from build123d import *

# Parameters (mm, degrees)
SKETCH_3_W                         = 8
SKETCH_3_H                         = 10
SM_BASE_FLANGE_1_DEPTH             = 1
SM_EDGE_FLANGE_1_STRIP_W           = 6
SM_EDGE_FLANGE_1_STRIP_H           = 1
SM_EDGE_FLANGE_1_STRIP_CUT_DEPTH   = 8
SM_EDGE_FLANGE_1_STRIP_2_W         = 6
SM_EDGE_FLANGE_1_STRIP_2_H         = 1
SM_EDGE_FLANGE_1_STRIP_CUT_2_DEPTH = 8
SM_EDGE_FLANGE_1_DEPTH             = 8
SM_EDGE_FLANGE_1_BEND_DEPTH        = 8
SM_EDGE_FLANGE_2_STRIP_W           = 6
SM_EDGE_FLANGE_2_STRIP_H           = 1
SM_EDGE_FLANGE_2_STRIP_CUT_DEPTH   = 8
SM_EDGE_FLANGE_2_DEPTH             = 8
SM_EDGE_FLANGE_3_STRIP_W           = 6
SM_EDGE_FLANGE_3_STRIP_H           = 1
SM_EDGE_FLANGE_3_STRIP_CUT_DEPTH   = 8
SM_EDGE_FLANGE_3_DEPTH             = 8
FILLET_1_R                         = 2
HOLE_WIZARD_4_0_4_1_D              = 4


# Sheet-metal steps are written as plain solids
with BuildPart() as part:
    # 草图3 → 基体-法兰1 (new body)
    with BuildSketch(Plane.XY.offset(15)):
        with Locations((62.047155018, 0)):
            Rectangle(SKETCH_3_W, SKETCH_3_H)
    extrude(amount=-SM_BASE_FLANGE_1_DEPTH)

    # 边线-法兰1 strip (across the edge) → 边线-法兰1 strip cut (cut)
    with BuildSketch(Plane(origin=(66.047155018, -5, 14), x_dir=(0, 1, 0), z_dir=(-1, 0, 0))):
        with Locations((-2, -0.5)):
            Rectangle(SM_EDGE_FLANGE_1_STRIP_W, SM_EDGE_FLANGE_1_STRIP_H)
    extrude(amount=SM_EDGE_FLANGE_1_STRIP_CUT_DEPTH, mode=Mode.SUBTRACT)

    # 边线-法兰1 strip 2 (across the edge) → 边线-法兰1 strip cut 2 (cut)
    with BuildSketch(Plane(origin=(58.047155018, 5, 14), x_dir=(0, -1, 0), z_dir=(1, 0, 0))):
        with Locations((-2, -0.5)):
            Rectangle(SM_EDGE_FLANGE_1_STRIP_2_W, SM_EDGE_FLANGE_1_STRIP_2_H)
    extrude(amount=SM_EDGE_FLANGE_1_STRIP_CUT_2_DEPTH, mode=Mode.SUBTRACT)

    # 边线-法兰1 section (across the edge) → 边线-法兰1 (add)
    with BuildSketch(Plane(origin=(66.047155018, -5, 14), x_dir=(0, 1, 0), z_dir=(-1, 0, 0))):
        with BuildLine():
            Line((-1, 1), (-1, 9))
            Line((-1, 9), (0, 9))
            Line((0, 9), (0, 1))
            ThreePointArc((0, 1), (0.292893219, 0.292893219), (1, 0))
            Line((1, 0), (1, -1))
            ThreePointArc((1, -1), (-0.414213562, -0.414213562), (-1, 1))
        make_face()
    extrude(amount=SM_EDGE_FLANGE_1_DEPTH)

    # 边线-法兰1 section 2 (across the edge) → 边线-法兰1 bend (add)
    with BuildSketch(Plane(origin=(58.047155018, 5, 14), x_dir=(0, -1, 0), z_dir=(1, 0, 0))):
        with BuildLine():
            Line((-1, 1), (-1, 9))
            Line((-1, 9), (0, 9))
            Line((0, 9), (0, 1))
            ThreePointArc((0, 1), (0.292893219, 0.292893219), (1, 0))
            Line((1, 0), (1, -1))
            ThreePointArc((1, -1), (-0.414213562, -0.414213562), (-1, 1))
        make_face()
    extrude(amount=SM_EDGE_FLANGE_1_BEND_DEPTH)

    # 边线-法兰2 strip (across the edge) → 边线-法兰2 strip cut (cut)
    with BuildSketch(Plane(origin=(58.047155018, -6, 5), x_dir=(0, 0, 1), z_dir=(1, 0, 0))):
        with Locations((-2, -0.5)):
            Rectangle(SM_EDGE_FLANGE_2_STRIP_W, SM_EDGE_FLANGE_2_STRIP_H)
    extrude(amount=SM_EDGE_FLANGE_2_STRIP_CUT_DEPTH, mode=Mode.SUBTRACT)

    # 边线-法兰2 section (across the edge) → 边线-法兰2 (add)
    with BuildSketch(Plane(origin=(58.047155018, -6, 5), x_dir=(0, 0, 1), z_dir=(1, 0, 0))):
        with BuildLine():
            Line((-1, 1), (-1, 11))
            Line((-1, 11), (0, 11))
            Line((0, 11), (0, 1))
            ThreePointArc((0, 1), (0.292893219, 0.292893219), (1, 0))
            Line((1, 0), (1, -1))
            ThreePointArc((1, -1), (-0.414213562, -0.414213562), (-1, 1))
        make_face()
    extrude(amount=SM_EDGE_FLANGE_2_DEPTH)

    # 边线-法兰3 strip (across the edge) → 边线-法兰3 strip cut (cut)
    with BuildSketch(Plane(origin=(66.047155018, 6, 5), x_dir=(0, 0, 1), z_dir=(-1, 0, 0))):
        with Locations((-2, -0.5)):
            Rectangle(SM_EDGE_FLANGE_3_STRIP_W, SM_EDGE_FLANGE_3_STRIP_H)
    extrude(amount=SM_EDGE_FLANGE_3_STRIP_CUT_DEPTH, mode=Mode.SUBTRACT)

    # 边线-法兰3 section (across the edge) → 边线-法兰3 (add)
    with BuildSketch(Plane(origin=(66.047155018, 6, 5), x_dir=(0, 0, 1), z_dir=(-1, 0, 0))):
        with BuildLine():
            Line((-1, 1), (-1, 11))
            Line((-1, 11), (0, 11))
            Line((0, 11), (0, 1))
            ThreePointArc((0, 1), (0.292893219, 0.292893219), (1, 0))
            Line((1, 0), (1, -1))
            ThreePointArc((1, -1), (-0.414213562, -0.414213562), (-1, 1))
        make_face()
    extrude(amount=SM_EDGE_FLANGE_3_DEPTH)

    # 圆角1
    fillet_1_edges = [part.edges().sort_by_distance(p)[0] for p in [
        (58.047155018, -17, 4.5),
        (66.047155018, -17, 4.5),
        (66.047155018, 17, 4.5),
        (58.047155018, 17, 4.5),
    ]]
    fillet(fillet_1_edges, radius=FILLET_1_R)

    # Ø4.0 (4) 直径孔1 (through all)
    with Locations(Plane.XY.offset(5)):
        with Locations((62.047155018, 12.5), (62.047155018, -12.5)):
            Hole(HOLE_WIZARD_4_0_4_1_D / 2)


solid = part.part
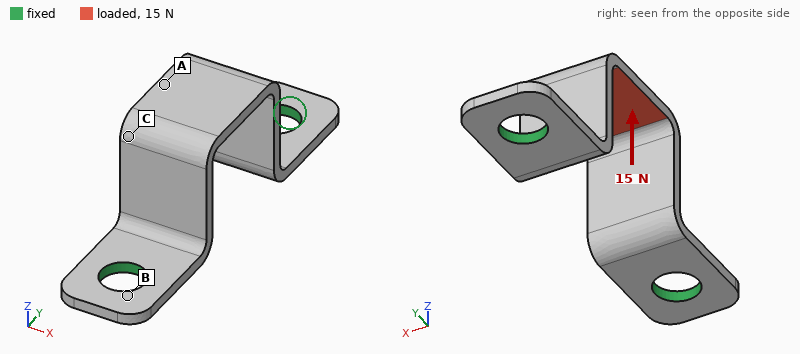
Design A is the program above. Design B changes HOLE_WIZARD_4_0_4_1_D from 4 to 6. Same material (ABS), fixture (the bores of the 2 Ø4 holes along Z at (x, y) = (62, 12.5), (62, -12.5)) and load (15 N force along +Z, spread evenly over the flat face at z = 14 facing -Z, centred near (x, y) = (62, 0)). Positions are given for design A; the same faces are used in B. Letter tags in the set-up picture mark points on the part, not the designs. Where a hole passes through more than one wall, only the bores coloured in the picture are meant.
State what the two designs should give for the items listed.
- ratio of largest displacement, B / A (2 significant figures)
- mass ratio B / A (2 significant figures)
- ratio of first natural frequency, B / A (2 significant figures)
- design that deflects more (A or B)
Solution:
0.76
0.92
1.2
A
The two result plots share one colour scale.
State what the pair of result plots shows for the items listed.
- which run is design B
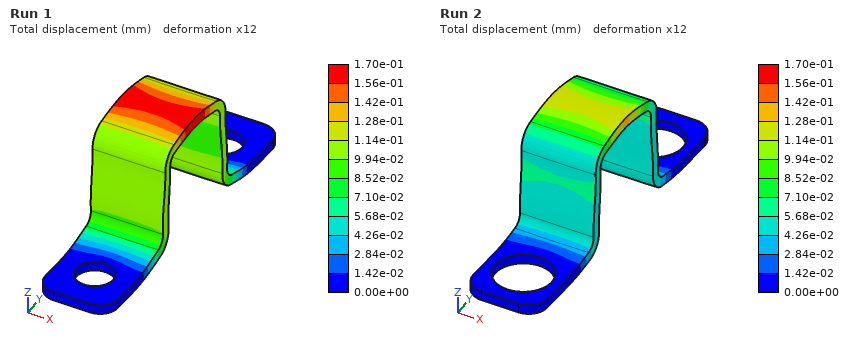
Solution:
Run 2
